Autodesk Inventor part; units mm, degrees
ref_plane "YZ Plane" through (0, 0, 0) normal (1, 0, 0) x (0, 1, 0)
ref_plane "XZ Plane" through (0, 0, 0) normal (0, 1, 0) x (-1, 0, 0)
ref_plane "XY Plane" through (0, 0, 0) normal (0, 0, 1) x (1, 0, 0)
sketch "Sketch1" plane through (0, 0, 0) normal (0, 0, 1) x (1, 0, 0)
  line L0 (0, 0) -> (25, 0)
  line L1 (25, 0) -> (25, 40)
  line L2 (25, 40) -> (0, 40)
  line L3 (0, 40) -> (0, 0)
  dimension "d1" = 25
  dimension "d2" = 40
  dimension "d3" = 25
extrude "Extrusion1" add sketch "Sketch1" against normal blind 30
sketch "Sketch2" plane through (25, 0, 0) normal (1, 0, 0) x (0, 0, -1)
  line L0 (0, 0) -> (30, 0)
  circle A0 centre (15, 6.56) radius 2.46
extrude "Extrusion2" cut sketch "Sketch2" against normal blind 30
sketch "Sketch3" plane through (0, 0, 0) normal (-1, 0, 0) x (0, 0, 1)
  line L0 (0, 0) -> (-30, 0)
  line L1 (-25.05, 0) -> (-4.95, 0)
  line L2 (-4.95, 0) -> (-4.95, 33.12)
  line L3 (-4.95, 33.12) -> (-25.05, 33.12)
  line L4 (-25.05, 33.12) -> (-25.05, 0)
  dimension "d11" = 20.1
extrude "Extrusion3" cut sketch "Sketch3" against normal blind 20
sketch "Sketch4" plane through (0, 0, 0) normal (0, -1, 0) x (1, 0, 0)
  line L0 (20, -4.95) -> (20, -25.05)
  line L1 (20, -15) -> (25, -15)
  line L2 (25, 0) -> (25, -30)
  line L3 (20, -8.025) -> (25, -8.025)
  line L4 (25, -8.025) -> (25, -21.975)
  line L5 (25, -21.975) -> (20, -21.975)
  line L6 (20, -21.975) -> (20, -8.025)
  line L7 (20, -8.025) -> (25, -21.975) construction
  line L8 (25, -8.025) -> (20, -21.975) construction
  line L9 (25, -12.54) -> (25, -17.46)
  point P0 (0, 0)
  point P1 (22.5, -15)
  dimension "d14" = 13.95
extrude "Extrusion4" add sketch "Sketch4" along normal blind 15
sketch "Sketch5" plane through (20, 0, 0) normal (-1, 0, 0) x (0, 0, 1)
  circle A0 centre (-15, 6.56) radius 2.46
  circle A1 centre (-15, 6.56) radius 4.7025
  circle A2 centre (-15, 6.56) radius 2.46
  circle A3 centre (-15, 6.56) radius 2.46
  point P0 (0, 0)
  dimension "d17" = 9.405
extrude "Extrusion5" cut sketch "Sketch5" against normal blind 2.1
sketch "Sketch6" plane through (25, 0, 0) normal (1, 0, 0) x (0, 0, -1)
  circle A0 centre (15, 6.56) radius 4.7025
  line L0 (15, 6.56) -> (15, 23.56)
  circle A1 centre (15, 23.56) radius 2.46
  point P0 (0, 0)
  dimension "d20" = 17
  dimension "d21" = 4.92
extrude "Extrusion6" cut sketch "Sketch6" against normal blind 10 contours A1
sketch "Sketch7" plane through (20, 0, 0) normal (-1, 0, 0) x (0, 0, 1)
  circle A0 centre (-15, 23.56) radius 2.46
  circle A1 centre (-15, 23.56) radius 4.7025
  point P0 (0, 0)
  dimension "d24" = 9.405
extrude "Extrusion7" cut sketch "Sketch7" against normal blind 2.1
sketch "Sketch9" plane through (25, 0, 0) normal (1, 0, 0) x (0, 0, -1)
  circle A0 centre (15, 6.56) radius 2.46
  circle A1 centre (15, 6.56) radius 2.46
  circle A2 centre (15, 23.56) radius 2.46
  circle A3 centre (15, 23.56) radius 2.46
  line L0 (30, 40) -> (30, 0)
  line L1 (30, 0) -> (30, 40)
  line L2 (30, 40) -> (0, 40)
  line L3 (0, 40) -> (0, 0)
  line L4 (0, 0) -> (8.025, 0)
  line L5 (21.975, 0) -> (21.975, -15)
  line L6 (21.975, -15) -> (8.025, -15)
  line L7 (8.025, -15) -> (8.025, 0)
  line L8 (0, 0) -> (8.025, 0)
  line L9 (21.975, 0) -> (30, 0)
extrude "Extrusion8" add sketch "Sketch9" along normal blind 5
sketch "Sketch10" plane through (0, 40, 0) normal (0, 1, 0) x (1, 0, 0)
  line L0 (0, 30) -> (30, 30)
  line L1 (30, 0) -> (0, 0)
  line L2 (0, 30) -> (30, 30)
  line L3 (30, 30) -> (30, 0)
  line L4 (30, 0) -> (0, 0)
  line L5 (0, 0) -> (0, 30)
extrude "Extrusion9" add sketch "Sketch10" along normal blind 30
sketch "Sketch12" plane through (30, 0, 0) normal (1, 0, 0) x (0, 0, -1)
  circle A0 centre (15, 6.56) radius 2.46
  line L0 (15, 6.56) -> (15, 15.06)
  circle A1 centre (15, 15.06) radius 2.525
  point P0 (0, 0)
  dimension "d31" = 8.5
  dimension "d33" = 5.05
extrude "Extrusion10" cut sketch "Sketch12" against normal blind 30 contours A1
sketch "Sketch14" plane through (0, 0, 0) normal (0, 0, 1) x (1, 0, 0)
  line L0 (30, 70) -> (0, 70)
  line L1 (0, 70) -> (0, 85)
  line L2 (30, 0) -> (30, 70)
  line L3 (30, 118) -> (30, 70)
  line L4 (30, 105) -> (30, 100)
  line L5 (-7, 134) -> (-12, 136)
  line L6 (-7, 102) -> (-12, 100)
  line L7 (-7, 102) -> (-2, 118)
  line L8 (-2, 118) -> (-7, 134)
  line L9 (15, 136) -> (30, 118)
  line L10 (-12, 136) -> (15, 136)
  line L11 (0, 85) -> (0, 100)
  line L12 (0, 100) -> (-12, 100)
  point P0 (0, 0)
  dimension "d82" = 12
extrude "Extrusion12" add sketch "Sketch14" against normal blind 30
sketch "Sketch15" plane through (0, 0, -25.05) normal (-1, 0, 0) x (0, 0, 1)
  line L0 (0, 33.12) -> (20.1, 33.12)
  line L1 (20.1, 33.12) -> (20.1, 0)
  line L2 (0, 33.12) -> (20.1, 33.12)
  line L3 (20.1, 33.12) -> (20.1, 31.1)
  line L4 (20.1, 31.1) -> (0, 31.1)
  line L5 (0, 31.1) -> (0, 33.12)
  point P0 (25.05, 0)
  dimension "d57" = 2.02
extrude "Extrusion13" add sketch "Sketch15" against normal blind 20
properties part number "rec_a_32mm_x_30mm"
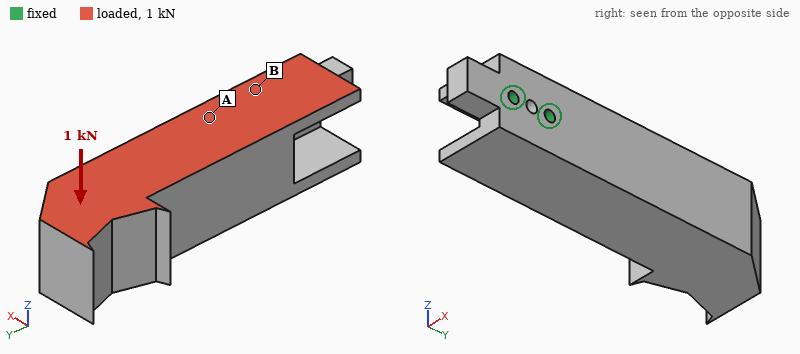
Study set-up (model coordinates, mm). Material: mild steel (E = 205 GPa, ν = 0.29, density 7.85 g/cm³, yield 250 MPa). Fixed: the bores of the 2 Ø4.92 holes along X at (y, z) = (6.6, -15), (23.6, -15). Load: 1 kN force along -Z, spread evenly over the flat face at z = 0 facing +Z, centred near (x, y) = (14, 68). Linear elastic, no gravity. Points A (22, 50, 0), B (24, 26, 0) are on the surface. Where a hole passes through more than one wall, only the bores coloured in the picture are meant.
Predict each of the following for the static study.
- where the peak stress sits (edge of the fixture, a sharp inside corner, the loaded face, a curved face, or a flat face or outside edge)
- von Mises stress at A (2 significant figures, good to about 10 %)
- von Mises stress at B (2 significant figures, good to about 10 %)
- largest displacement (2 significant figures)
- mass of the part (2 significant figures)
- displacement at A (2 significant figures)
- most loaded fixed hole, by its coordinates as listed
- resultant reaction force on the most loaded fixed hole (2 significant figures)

edge of the fixture
6.6 MPa
20 MPa
39 µm
880 g
8.4 µm
(23.6, -15)
2.9 kN
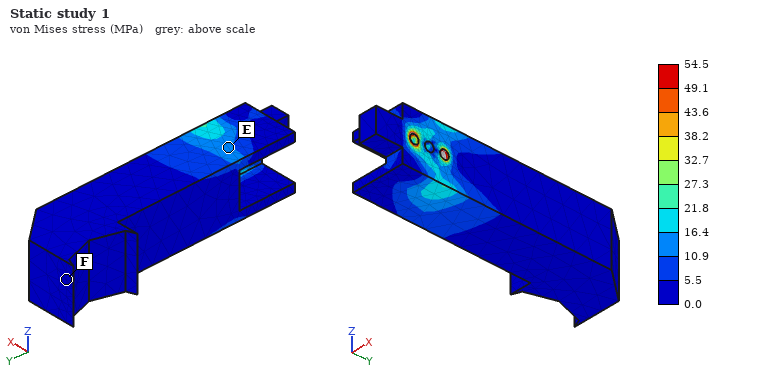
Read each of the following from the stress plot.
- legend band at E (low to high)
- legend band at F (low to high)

10.9 to 16.4 MPa
0.0 to 5.5 MPa
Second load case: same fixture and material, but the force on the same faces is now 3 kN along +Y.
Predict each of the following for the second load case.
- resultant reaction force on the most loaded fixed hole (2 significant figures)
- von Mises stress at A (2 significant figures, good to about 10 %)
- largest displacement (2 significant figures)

3.0 kN
9.8 MPa
46 µm
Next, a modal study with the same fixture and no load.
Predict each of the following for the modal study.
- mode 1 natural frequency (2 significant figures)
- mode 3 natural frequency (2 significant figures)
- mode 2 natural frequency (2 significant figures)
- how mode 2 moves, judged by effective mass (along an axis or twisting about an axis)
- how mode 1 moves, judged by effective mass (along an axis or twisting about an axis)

890 Hz
3000 Hz
1000 Hz
along Z
along X
